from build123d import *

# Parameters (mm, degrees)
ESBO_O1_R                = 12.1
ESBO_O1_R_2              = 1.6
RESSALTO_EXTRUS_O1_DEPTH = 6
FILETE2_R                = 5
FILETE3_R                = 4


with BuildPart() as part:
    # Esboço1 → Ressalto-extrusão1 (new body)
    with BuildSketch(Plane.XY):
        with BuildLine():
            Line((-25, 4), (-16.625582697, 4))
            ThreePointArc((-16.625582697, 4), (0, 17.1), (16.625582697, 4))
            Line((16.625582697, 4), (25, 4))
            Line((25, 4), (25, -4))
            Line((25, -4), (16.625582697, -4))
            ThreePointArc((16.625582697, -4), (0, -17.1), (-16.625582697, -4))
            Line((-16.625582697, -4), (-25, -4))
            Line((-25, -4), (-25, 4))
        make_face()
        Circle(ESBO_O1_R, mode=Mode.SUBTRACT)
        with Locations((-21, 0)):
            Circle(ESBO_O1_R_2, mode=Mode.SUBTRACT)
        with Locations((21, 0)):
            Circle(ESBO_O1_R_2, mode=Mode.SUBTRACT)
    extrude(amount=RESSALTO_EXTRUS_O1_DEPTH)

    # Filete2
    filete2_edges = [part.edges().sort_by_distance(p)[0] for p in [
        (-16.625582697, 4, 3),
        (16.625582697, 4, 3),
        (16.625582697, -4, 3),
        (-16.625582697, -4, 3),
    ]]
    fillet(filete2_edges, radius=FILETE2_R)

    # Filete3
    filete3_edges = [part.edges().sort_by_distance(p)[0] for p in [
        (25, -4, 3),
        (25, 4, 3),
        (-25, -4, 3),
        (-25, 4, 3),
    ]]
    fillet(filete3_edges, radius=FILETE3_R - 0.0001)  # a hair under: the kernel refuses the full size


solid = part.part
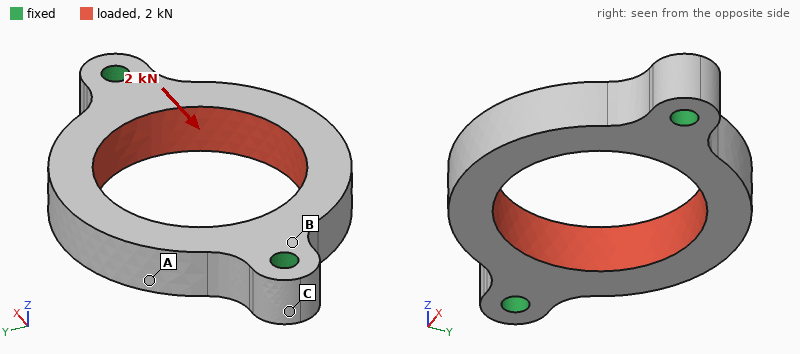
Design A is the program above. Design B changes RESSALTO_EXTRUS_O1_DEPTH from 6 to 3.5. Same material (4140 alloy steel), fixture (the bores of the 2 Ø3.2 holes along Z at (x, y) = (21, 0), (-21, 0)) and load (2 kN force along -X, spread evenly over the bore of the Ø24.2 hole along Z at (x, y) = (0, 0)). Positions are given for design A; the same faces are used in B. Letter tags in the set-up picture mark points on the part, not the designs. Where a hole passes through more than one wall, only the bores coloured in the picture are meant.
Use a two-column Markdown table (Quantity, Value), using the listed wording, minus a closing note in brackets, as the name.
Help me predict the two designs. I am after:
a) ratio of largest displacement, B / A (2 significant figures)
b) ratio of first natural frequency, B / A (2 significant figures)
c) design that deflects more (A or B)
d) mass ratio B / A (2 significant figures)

| Quantity | Value |
|---|---|
| ratio of largest displacement, B / A | 1.7 |
| ratio of first natural frequency, B / A | 0.65 |
| design that deflects more | B |
| mass ratio B / A | 0.58 |
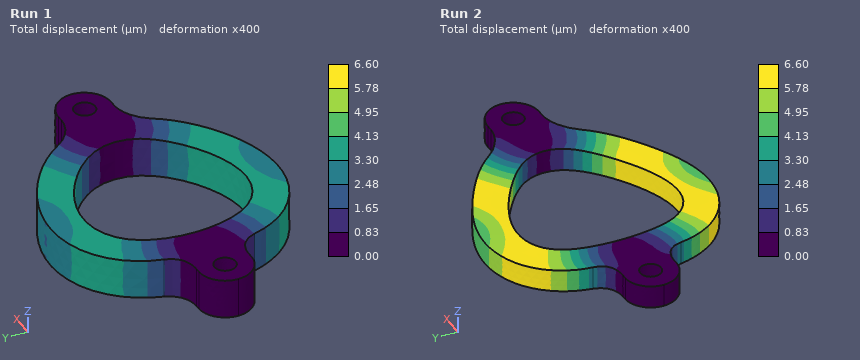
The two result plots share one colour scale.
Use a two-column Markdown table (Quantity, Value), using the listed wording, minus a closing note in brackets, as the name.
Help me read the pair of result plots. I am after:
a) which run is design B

| Quantity | Value |
|---|---|
| which run is design B | Run 2 |
